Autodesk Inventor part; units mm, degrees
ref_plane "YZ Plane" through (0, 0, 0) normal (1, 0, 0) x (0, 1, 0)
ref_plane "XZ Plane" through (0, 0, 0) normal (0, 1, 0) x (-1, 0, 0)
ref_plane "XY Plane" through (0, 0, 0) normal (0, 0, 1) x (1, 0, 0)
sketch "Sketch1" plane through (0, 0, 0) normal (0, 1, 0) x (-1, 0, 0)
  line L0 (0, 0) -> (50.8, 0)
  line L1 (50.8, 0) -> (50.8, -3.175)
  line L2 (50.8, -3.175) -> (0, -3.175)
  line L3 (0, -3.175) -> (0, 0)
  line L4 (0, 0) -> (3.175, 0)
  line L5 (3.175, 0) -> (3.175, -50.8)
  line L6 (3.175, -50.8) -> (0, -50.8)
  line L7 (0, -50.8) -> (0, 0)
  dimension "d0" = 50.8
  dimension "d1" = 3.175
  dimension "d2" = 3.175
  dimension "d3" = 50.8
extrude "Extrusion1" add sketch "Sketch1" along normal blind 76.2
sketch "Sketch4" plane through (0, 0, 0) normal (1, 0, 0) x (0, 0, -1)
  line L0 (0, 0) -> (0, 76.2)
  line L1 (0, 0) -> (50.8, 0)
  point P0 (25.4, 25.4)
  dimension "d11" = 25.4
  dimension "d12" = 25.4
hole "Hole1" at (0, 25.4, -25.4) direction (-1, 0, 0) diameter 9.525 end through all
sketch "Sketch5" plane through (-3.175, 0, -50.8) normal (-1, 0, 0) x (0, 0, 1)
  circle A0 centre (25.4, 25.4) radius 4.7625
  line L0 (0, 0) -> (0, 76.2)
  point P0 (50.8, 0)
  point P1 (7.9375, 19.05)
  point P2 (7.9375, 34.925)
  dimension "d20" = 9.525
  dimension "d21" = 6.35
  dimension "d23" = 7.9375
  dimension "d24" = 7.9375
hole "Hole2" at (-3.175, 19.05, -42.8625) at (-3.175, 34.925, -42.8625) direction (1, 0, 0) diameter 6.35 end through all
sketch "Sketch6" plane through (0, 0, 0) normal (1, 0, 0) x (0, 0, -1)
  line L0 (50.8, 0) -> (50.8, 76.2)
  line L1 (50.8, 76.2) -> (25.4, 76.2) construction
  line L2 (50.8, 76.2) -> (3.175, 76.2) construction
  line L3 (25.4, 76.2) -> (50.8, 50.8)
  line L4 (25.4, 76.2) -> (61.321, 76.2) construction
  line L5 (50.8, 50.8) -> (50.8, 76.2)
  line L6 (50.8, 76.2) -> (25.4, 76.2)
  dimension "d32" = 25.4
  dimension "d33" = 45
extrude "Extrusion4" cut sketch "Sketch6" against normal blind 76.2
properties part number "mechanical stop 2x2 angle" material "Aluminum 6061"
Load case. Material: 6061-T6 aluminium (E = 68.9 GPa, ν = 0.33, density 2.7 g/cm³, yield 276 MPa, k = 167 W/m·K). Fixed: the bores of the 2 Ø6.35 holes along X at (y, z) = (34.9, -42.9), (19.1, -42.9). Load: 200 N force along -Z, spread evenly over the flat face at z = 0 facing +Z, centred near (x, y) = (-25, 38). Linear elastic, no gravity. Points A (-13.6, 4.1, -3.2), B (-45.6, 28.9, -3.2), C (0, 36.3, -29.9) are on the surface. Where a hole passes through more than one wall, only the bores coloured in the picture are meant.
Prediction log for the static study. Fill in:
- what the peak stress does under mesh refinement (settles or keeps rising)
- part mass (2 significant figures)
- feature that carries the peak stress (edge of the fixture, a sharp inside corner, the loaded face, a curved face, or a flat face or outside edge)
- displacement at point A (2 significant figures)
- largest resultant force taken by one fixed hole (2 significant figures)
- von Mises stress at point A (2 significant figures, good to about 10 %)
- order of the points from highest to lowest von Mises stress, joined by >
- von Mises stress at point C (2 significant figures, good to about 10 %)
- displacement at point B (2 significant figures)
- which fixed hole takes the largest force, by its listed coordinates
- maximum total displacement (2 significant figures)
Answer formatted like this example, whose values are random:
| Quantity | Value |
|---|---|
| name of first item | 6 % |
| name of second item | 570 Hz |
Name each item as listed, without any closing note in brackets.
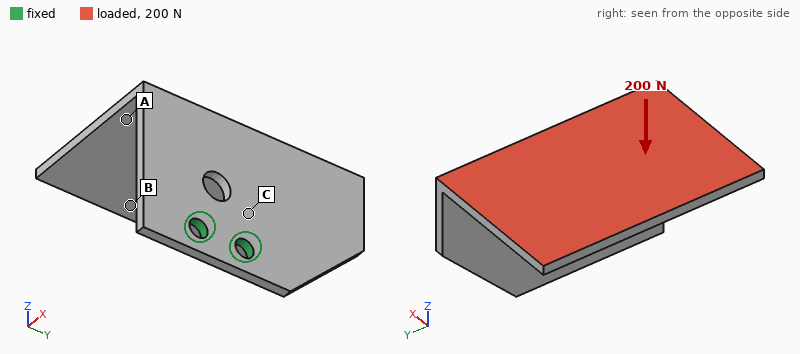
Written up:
| Quantity | Value |
|---|---|
| what the peak stress does under mesh refinement | keeps rising |
| part mass | 60 g |
| feature that carries the peak stress | edge of the fixture |
| displacement at point A | 0.36 mm |
| largest resultant force taken by one fixed hole | 200 N |
| von Mises stress at point A | 21 MPa |
| order of the points from highest to lowest von Mises stress, joined by > | C > A > B |
| von Mises stress at point C | 48 MPa |
| displacement at point B | 0.91 mm |
| which fixed hole takes the largest force, by its listed coordinates | (34.9, -42.9) |
| maximum total displacement | 1.1 mm |
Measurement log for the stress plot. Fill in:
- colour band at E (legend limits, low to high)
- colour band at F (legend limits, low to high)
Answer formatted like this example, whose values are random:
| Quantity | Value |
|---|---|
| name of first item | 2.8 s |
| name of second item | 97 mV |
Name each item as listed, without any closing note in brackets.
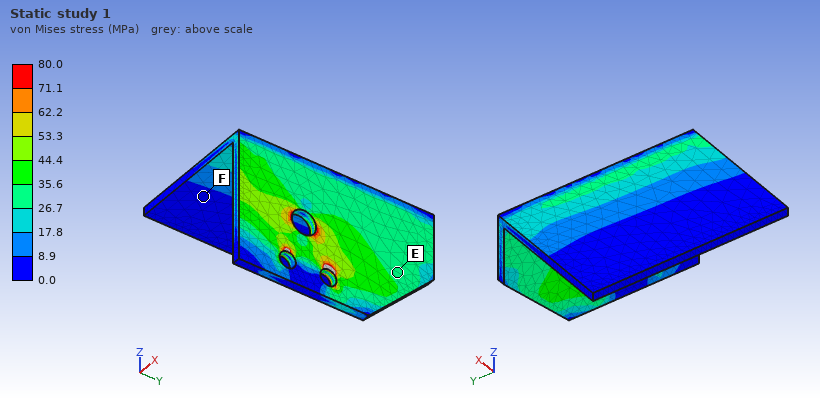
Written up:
| Quantity | Value |
|---|---|
| colour band at E | 26.7 to 35.6 MPa |
| colour band at F | 0.0 to 8.9 MPa |
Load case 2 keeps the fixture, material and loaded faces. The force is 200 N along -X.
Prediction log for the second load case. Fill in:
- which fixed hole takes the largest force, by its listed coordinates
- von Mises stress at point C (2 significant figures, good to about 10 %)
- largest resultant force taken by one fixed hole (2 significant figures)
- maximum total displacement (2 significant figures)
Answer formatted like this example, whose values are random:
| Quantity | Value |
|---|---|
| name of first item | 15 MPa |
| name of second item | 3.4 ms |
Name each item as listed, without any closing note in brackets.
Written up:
| Quantity | Value |
|---|---|
| which fixed hole takes the largest force, by its listed coordinates | (34.9, -42.9) |
| von Mises stress at point C | 70 MPa |
| largest resultant force taken by one fixed hole | 180 N |
| maximum total displacement | 1.1 mm |
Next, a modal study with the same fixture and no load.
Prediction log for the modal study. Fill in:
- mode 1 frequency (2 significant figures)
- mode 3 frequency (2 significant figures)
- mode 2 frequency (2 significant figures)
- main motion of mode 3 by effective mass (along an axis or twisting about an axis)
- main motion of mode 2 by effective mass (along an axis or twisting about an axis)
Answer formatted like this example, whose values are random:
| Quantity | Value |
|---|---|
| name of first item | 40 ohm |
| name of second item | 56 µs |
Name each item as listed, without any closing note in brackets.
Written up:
| Quantity | Value |
|---|---|
| mode 1 frequency | 380 Hz |
| mode 3 frequency | 1100 Hz |
| mode 2 frequency | 580 Hz |
| main motion of mode 3 by effective mass | along X |
| main motion of mode 2 by effective mass | along Y |
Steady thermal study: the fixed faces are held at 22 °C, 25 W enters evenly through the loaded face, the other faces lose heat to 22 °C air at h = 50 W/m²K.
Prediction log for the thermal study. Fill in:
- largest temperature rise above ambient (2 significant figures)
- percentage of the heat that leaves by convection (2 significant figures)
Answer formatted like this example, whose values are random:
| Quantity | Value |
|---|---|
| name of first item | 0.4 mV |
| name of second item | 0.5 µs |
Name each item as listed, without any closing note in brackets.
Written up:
| Quantity | Value |
|---|---|
| largest temperature rise above ambient | 32 K |
| percentage of the heat that leaves by convection | 41 % |
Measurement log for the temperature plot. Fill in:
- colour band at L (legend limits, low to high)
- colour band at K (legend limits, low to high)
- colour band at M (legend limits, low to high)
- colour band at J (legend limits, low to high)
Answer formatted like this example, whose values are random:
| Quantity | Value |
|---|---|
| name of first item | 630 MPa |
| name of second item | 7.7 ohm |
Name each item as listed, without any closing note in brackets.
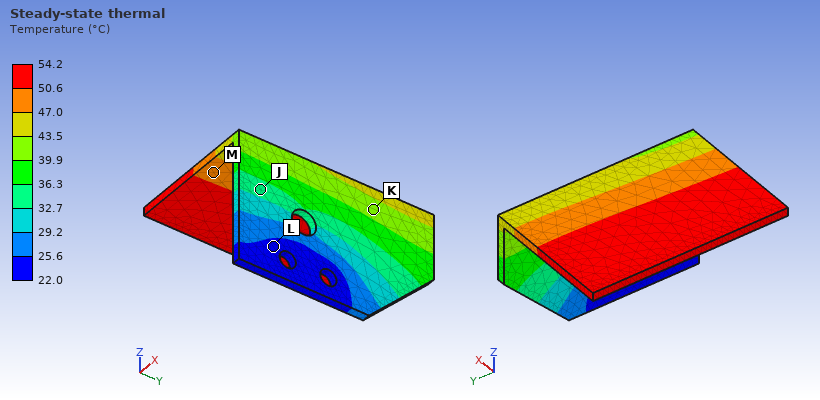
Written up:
| Quantity | Value |
|---|---|
| colour band at L | 22.0 to 25.6 °C |
| colour band at K | 39.9 to 43.5 °C |
| colour band at M | 47.0 to 50.6 °C |
| colour band at J | 32.7 to 36.3 °C |
